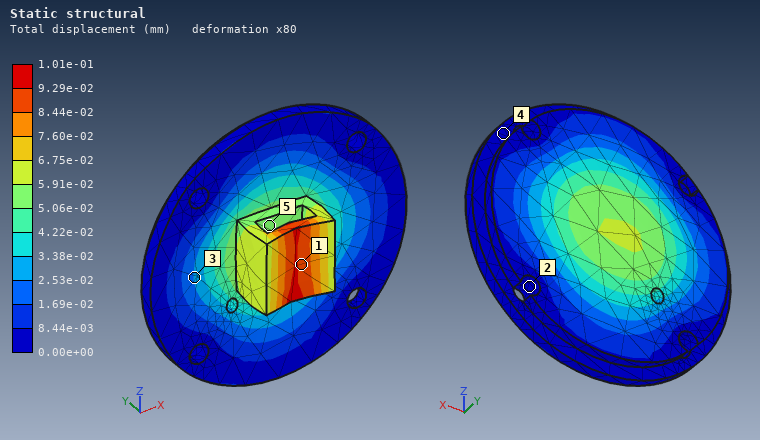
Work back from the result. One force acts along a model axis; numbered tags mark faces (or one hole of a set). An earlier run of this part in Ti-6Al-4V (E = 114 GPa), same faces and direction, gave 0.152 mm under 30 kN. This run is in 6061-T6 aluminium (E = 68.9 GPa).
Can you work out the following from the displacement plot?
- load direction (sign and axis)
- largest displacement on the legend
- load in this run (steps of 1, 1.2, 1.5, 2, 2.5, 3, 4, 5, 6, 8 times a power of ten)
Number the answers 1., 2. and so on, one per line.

1. +Y
2. 1.01e-01 mm
3. 12 kN
